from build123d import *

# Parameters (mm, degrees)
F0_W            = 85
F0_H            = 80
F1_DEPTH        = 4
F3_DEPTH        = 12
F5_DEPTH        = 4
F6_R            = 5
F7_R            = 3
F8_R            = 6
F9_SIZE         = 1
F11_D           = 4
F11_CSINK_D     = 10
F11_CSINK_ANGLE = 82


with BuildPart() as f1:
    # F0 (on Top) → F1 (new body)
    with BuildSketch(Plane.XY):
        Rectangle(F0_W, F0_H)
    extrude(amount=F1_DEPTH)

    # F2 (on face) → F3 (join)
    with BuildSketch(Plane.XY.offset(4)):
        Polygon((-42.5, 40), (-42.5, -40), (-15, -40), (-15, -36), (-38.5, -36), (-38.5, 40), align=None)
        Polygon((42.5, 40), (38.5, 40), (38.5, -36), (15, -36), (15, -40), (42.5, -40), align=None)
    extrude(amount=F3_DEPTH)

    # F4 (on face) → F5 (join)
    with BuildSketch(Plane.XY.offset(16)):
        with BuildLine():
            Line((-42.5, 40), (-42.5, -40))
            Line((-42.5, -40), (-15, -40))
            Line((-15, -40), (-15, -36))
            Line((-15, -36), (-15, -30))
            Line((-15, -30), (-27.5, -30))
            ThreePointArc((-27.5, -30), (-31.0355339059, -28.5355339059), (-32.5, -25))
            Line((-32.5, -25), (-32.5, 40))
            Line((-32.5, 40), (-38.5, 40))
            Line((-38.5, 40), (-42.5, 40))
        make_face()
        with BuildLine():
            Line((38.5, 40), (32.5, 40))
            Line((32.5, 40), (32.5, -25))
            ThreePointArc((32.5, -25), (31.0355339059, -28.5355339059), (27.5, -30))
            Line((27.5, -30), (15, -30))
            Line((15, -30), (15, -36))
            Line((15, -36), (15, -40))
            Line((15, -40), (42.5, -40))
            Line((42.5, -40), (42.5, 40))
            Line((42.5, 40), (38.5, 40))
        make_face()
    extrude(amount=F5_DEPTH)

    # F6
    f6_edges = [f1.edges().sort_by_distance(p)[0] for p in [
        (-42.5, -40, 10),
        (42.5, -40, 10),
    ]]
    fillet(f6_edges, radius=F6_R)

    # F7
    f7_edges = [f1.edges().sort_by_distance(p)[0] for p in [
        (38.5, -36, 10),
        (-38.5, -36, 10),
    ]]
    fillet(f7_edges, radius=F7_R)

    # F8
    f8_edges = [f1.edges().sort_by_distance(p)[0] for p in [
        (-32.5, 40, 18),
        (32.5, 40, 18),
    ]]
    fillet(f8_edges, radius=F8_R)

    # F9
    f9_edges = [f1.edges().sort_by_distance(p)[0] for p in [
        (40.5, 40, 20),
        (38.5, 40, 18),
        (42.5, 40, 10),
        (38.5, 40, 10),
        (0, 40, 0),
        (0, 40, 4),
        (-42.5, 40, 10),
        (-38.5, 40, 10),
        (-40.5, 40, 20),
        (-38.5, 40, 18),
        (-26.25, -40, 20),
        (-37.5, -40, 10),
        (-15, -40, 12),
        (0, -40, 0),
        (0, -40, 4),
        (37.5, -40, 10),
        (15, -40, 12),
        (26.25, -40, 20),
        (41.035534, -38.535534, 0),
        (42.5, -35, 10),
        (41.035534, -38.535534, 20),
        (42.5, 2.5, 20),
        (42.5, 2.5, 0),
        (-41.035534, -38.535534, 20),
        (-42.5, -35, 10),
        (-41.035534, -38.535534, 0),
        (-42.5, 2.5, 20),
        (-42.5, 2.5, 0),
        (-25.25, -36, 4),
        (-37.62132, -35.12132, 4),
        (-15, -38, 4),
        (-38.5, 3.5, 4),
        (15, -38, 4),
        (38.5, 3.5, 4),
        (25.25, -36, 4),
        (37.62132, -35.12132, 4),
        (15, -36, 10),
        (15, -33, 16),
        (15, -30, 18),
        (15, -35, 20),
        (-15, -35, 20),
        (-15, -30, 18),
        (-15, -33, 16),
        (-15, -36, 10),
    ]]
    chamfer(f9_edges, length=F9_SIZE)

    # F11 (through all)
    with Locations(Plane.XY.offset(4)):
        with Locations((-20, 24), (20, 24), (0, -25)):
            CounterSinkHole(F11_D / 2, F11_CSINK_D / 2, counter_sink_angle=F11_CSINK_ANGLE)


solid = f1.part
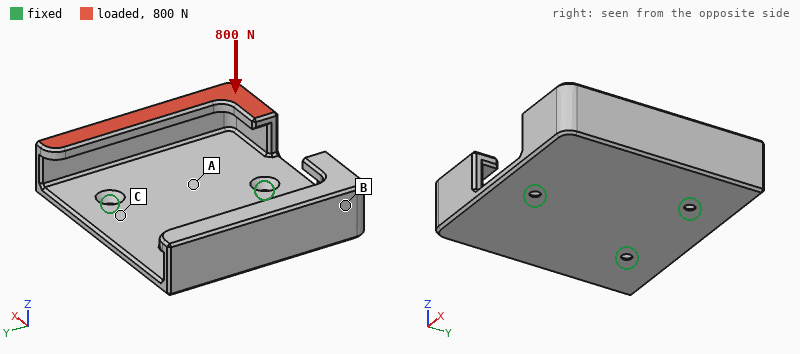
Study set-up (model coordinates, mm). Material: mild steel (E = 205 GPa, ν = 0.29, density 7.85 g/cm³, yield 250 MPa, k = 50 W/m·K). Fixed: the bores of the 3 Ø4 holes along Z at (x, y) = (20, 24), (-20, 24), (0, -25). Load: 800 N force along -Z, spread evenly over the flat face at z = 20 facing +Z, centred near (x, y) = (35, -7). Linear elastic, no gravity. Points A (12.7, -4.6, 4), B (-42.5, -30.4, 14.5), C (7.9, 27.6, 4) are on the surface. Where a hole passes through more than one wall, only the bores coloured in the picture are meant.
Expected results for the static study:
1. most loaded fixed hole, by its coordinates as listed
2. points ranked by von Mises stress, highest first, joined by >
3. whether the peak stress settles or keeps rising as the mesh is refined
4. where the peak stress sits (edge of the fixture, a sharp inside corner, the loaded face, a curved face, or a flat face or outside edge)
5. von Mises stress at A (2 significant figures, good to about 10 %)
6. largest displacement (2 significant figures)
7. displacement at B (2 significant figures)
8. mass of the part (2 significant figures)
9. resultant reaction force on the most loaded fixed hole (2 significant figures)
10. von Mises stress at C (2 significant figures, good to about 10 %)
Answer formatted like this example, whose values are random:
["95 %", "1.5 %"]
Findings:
["(-20, 24)", "A > C > B", "keeps rising", "edge of the fixture", "68 MPa", "0.24 mm", "0.057 mm", "340 g", "1.5 kN", "41 MPa"]
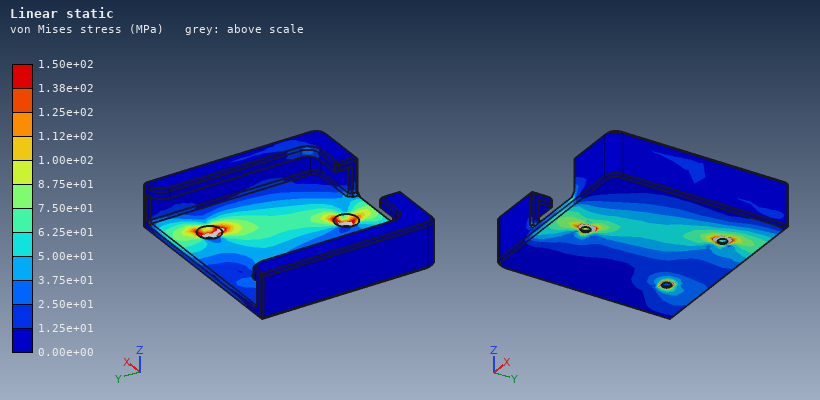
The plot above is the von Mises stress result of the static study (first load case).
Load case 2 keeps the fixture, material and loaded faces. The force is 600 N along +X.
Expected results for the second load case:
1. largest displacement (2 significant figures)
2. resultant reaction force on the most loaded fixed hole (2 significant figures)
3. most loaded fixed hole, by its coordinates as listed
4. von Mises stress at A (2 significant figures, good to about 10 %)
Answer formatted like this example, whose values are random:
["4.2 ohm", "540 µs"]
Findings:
["0.15 mm", "900 N", "(-20, 24)", "41 MPa"]
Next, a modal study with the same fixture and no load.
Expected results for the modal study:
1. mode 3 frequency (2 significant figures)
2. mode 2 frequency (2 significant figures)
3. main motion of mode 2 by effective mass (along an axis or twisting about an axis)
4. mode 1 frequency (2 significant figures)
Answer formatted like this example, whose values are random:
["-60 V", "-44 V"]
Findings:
["2500 Hz", "1200 Hz", "along Z", "910 Hz"]
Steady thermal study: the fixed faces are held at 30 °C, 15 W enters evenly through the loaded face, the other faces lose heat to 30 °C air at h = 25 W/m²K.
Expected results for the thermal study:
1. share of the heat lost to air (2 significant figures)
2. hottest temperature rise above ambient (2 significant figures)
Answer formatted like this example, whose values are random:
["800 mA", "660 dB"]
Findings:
["47 %", "37 K"]
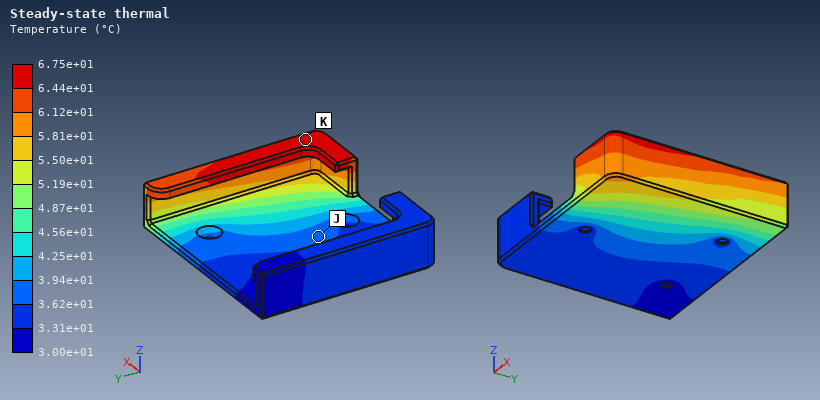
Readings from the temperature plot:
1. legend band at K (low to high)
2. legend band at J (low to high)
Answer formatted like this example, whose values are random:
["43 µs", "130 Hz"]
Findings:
["6.44e+01 to 6.75e+01 °C", "3.62e+01 to 3.94e+01 °C"]
